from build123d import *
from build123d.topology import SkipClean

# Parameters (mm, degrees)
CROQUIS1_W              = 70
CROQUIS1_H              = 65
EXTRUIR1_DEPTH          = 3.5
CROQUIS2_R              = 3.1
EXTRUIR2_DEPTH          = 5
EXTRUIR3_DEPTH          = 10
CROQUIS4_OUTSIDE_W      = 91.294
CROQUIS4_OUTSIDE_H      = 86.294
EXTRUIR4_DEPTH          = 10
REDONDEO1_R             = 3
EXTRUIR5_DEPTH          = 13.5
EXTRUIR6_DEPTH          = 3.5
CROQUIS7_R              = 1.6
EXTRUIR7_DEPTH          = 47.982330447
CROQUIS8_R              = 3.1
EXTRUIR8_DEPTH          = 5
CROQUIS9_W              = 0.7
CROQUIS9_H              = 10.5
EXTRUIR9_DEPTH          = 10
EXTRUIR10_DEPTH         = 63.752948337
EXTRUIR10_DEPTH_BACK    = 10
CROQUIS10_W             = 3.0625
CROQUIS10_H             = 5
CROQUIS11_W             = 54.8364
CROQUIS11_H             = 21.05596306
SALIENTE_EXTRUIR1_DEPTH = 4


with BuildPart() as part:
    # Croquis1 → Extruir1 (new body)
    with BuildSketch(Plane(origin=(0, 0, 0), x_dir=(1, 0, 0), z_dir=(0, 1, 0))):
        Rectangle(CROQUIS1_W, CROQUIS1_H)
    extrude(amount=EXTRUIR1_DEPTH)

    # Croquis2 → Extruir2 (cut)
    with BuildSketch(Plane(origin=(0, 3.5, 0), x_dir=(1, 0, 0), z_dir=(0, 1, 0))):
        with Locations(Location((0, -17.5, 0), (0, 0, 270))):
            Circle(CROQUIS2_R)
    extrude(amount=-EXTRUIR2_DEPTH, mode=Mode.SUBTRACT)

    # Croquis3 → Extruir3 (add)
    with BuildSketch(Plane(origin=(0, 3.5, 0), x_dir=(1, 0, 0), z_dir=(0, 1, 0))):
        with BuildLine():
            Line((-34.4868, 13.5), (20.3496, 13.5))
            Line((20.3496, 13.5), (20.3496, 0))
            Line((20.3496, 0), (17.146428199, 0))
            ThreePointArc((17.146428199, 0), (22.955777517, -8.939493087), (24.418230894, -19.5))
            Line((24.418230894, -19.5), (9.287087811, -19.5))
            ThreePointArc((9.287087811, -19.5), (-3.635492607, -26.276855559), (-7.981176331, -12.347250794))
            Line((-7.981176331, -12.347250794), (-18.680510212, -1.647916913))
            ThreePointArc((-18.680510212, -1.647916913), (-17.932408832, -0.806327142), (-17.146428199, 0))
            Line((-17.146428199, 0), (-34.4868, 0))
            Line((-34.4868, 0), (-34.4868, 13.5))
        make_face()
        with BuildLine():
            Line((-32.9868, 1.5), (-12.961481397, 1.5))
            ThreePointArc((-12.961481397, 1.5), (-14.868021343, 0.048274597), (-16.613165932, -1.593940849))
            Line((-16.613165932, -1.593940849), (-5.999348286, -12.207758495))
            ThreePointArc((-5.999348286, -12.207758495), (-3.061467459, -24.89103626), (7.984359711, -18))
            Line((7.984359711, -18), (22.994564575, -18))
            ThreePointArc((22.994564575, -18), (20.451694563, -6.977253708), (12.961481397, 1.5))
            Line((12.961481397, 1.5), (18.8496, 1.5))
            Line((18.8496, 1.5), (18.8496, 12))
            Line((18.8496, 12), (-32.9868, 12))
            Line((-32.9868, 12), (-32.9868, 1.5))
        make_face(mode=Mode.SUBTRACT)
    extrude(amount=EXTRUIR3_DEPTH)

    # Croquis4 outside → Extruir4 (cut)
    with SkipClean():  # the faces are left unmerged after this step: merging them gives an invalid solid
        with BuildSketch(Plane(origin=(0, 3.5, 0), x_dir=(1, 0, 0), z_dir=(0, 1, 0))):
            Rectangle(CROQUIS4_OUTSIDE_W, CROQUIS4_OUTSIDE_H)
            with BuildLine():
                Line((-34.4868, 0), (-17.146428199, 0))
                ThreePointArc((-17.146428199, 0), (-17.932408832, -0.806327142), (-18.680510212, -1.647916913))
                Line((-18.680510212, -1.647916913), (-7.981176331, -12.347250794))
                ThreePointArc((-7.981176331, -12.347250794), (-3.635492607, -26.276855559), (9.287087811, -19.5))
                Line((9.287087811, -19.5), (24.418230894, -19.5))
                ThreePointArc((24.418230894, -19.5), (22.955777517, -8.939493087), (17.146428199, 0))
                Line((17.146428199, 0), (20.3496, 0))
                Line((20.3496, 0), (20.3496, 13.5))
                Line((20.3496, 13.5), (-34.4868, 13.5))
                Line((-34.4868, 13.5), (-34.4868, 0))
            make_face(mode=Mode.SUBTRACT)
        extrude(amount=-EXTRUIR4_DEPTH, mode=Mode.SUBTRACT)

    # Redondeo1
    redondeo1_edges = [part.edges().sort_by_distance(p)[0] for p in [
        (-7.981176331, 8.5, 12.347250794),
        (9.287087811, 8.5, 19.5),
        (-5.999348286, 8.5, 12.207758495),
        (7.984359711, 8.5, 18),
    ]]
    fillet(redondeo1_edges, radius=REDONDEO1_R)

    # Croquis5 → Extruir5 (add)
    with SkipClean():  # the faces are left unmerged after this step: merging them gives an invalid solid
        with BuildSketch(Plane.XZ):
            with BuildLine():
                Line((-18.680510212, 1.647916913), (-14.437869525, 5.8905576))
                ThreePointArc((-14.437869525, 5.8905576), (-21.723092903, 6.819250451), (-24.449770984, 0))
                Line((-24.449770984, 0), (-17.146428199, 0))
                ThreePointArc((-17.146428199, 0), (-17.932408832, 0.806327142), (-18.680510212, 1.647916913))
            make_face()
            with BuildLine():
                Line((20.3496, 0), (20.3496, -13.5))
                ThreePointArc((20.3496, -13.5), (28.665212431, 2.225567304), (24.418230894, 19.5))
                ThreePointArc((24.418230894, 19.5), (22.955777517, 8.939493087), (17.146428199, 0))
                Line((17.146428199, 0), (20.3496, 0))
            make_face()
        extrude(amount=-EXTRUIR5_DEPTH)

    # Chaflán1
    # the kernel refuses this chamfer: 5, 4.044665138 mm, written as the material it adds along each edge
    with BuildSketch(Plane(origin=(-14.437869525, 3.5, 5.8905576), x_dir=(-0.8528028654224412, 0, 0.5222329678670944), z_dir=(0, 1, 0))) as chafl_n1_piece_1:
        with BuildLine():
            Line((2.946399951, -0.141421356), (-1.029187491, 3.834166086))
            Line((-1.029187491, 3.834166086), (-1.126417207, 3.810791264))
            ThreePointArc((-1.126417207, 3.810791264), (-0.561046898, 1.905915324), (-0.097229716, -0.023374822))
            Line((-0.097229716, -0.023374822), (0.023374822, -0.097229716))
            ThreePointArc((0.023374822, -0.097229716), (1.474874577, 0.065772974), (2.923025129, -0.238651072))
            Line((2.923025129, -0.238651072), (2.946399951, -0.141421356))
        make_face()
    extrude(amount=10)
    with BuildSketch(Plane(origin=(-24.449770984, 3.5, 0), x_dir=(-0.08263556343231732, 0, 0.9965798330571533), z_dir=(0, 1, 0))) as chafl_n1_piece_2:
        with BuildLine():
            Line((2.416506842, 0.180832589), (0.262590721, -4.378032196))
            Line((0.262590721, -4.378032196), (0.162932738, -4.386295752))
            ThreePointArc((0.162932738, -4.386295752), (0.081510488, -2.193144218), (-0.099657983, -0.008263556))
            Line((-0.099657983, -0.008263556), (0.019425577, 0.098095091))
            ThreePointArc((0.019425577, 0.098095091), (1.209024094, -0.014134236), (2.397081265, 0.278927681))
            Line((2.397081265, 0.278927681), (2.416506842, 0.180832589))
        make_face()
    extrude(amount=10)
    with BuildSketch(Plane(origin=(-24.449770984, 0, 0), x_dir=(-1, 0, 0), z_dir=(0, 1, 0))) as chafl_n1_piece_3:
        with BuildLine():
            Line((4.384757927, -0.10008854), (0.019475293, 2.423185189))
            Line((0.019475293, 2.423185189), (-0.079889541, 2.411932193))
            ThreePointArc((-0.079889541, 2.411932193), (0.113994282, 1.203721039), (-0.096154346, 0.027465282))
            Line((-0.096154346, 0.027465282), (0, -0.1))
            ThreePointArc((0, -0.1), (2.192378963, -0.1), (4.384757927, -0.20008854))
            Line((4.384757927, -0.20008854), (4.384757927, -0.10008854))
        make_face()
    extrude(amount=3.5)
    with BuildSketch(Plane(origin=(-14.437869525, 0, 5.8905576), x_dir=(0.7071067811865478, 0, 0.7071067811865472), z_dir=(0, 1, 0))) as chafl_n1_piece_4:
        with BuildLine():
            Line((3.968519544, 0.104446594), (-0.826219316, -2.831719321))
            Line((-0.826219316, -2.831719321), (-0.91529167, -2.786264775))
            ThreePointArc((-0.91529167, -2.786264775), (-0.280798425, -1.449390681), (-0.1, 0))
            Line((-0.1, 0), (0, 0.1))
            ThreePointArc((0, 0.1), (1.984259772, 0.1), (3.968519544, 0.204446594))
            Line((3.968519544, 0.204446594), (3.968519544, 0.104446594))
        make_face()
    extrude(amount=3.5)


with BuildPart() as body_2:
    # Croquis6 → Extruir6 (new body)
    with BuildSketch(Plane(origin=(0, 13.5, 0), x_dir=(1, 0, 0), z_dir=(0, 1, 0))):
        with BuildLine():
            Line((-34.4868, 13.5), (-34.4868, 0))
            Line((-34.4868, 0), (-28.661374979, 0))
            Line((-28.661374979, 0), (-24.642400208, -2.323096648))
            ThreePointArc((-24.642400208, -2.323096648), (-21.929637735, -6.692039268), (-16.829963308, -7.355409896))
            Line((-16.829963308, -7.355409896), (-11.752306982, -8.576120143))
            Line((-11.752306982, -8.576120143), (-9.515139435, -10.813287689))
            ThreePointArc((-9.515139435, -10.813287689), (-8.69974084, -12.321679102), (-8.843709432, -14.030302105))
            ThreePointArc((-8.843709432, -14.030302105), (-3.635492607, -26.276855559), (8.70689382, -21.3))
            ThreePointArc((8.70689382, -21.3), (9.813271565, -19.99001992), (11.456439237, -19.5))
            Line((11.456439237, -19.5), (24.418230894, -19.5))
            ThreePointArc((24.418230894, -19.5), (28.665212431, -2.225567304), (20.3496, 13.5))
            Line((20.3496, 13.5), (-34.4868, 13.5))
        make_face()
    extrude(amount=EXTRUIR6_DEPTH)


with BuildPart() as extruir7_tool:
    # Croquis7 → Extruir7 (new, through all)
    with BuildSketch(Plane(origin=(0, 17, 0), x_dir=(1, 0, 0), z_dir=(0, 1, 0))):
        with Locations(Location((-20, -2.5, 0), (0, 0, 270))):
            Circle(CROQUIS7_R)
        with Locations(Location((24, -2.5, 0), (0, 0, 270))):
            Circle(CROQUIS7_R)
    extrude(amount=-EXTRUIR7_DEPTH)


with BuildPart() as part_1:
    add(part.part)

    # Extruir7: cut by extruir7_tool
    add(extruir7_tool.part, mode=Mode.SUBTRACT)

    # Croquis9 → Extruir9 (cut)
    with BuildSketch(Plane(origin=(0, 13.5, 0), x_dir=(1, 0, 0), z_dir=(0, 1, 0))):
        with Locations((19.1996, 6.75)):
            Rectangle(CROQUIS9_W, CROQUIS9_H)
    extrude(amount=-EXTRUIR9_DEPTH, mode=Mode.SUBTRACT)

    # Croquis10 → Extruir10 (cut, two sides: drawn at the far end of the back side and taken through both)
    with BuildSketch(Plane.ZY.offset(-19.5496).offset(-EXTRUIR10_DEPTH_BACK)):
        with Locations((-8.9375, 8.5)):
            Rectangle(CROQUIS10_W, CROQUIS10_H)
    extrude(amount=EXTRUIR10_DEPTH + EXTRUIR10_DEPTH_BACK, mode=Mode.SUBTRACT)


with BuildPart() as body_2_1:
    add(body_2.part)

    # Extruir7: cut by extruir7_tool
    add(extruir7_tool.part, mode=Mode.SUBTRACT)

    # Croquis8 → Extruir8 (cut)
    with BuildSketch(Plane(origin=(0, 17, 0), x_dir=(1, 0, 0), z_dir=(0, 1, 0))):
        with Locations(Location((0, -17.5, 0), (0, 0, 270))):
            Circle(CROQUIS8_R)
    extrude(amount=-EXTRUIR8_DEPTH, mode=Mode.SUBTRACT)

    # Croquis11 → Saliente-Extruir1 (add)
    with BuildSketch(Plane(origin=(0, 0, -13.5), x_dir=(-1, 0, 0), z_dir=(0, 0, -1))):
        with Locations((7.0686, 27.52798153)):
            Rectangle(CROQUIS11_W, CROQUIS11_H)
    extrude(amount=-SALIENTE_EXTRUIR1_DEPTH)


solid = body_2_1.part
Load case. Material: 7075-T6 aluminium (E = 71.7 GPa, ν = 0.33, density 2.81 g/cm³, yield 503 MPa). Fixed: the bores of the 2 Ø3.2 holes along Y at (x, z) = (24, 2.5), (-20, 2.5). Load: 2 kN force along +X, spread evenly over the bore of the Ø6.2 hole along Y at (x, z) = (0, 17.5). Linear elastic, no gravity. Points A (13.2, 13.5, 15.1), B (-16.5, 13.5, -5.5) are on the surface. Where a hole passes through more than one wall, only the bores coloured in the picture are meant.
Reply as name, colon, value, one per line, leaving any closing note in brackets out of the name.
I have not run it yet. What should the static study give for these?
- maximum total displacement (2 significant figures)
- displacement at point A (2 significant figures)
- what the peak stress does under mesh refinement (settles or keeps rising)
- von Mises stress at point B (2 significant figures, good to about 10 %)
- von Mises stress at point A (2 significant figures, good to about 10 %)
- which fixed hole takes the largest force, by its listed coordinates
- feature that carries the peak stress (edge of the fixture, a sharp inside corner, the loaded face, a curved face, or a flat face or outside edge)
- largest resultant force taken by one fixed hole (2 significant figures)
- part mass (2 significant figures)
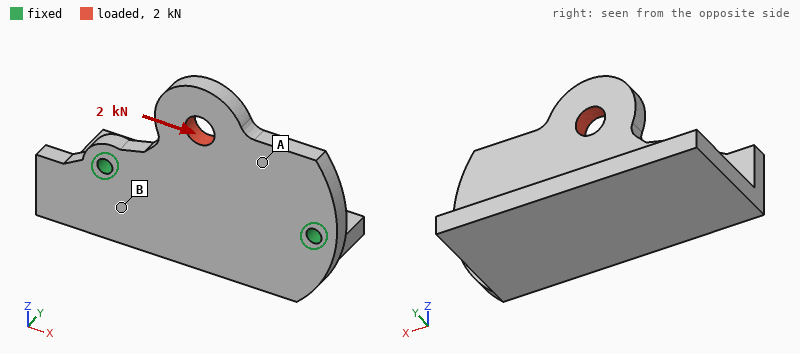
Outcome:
maximum total displacement: 24 µm
displacement at point A: 11 µm
what the peak stress does under mesh refinement: keeps rising
von Mises stress at point B: 11 MPa
von Mises stress at point A: 32 MPa
which fixed hole takes the largest force, by its listed coordinates: (24, 2.5)
feature that carries the peak stress: edge of the fixture
largest resultant force taken by one fixed hole: 1.4 kN
part mass: 30 g
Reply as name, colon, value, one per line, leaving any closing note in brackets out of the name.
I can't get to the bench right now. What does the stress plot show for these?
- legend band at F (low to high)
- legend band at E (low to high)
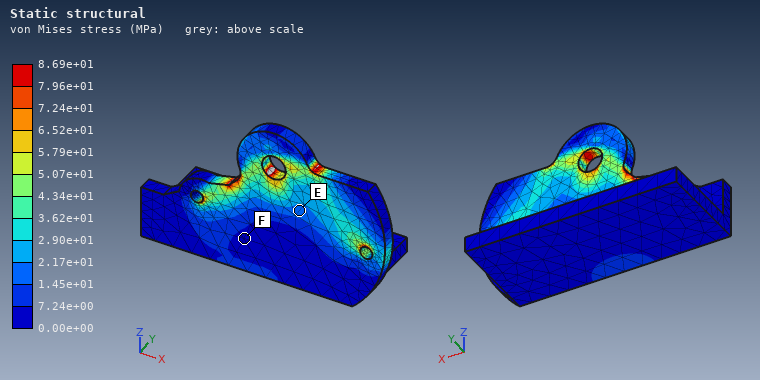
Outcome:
legend band at F: 0.00e+00 to 7.24e+00 MPa
legend band at E: 1.45e+01 to 2.17e+01 MPa
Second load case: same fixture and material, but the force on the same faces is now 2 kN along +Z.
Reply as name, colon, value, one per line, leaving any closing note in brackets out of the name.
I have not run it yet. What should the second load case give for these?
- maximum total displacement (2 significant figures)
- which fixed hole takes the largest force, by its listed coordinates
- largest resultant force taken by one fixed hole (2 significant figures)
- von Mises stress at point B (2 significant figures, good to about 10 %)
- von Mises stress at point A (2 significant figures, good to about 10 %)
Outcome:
maximum total displacement: 20 µm
which fixed hole takes the largest force, by its listed coordinates: (-20, 2.5)
largest resultant force taken by one fixed hole: 1.1 kN
von Mises stress at point B: 23 MPa
von Mises stress at point A: 11 MPa
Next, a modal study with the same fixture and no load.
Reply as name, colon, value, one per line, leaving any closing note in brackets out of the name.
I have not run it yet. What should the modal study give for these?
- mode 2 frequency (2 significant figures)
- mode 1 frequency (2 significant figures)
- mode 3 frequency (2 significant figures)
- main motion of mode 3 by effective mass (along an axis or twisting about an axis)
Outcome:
mode 2 frequency: 4400 Hz
mode 1 frequency: 2200 Hz
mode 3 frequency: 4900 Hz
main motion of mode 3 by effective mass: along Y
